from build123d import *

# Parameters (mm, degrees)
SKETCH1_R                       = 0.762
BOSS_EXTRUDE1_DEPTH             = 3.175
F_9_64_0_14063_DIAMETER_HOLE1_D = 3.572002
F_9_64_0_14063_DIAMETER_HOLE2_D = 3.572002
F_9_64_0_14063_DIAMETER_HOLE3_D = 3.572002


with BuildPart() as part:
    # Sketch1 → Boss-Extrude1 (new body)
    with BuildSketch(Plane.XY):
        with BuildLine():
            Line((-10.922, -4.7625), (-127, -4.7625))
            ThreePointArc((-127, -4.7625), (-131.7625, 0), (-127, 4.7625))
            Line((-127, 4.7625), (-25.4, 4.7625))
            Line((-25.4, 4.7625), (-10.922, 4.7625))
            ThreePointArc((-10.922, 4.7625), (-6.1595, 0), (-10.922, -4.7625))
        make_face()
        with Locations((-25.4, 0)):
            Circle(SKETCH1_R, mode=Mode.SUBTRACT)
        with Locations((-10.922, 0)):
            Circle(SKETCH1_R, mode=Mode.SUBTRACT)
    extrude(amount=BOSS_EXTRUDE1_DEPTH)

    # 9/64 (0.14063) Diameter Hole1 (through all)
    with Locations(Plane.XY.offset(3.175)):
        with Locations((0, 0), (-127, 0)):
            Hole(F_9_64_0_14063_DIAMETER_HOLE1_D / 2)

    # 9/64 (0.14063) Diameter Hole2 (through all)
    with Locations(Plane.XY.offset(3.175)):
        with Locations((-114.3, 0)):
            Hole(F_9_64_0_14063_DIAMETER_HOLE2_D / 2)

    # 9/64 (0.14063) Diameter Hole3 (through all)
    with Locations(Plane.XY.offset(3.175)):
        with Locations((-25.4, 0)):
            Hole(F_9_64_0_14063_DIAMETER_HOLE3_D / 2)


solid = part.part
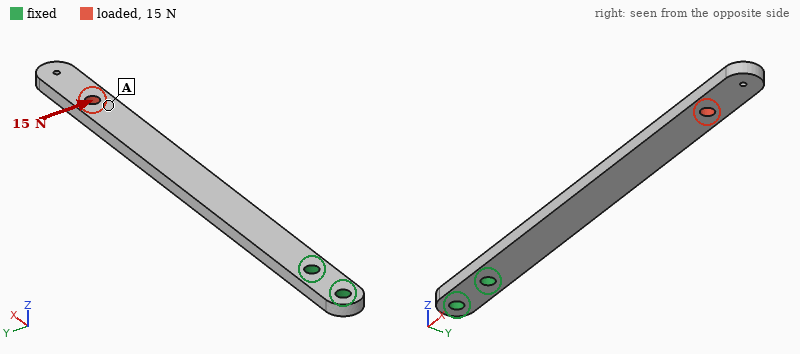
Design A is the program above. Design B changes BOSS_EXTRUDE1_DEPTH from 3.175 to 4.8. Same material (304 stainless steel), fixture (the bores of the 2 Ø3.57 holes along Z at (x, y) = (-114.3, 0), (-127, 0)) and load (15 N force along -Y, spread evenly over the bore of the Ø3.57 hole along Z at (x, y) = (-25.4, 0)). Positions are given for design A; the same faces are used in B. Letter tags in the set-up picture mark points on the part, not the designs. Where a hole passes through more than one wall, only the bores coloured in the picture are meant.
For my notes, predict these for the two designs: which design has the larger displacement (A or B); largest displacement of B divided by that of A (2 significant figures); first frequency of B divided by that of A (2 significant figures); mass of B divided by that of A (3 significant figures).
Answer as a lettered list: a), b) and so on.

a) A
b) 0.66
c) 1.5
d) 1.51
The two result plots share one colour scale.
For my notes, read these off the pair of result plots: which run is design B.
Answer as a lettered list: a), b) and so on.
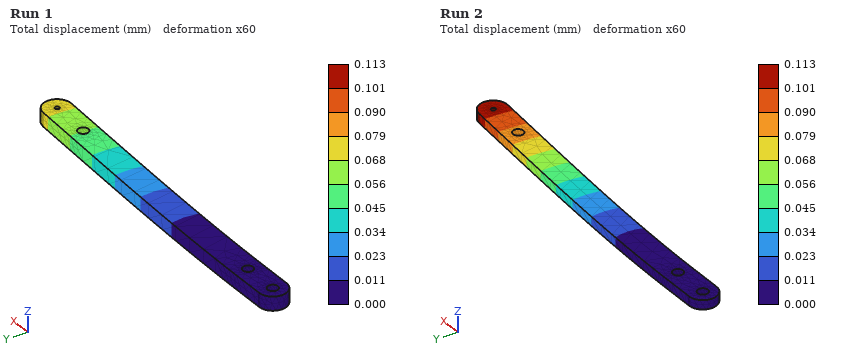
a) Run 1
